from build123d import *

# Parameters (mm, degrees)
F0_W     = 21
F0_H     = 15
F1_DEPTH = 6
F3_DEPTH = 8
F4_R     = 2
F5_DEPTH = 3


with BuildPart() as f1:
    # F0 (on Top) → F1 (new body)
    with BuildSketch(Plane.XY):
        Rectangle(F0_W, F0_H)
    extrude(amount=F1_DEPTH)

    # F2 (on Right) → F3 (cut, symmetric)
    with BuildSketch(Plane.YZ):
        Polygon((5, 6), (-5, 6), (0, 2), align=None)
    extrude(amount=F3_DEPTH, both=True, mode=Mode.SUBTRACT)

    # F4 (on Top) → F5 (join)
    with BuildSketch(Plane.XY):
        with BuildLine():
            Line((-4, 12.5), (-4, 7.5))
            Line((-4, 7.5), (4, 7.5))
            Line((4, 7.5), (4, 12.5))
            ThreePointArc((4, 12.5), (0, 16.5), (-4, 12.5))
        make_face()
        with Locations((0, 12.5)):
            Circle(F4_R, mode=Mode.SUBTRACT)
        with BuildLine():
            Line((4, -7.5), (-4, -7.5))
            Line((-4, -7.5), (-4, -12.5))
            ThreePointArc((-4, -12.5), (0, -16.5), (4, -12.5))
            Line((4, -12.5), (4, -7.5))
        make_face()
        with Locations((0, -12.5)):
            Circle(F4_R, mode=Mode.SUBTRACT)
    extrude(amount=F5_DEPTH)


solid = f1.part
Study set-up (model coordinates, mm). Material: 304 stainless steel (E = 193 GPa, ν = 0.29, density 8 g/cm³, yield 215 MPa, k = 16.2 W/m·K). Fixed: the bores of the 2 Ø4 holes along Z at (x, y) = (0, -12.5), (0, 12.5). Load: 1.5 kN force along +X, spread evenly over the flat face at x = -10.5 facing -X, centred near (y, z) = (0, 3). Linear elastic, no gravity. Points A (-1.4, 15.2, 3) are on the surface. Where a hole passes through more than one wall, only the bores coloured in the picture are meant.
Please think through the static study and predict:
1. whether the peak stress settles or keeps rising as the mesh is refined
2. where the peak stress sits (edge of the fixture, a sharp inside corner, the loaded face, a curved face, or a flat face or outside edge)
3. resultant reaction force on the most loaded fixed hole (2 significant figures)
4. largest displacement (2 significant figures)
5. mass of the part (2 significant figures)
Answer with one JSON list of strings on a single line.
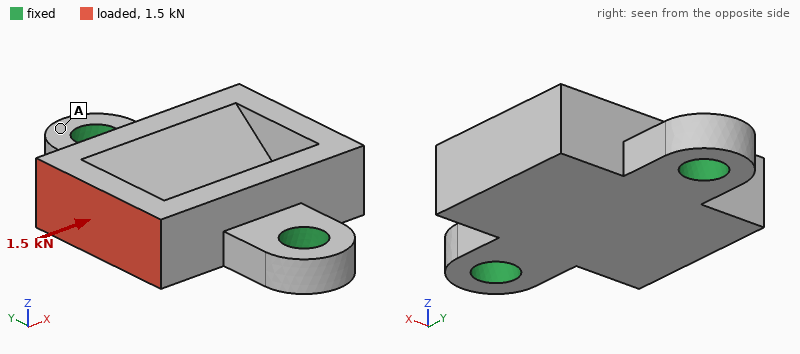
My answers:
["keeps rising", "edge of the fixture", "750 N", "16 µm", "15 g"]
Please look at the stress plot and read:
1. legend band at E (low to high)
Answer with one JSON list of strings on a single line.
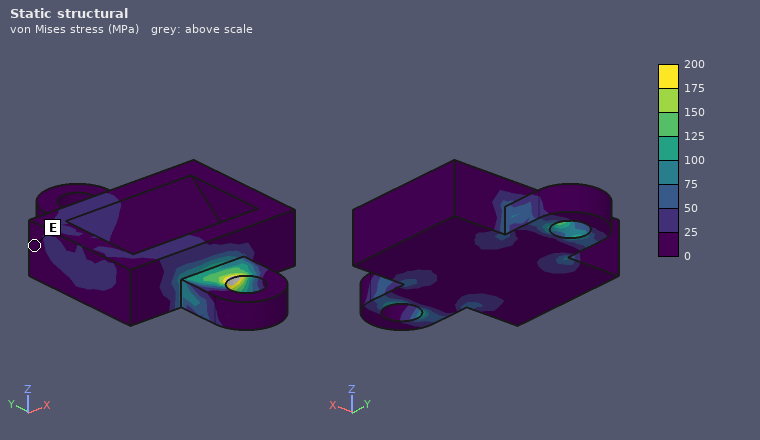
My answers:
["0 to 25 MPa"]
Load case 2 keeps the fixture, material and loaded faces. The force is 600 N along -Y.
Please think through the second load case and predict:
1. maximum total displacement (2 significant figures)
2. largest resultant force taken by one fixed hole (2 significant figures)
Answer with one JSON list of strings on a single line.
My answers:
["3.8 µm", "420 N"]
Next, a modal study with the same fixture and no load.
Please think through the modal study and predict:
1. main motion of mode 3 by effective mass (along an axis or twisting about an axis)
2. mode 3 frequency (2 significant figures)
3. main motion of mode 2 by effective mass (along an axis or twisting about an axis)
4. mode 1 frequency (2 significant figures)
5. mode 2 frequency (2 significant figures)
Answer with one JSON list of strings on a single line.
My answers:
["along X", "31 kHz", "along Z", "10 kHz", "17 kHz"]
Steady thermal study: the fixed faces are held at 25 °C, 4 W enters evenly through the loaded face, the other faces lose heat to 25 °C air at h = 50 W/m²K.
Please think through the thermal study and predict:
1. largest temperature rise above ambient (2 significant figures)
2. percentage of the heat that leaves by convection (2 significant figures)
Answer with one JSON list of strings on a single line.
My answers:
["50 K", "30 %"]
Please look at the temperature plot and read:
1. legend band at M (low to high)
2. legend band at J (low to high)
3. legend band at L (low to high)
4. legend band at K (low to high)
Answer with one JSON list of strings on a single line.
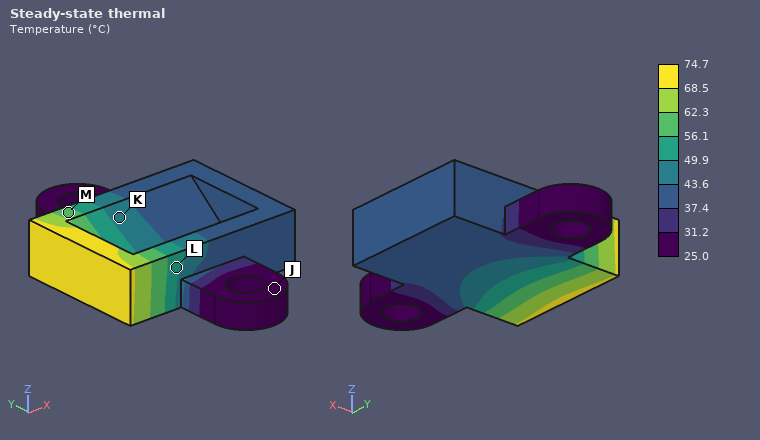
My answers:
["56.1 to 62.3 °C", "25.0 to 31.2 °C", "49.9 to 56.1 °C", "43.6 to 49.9 °C"]
